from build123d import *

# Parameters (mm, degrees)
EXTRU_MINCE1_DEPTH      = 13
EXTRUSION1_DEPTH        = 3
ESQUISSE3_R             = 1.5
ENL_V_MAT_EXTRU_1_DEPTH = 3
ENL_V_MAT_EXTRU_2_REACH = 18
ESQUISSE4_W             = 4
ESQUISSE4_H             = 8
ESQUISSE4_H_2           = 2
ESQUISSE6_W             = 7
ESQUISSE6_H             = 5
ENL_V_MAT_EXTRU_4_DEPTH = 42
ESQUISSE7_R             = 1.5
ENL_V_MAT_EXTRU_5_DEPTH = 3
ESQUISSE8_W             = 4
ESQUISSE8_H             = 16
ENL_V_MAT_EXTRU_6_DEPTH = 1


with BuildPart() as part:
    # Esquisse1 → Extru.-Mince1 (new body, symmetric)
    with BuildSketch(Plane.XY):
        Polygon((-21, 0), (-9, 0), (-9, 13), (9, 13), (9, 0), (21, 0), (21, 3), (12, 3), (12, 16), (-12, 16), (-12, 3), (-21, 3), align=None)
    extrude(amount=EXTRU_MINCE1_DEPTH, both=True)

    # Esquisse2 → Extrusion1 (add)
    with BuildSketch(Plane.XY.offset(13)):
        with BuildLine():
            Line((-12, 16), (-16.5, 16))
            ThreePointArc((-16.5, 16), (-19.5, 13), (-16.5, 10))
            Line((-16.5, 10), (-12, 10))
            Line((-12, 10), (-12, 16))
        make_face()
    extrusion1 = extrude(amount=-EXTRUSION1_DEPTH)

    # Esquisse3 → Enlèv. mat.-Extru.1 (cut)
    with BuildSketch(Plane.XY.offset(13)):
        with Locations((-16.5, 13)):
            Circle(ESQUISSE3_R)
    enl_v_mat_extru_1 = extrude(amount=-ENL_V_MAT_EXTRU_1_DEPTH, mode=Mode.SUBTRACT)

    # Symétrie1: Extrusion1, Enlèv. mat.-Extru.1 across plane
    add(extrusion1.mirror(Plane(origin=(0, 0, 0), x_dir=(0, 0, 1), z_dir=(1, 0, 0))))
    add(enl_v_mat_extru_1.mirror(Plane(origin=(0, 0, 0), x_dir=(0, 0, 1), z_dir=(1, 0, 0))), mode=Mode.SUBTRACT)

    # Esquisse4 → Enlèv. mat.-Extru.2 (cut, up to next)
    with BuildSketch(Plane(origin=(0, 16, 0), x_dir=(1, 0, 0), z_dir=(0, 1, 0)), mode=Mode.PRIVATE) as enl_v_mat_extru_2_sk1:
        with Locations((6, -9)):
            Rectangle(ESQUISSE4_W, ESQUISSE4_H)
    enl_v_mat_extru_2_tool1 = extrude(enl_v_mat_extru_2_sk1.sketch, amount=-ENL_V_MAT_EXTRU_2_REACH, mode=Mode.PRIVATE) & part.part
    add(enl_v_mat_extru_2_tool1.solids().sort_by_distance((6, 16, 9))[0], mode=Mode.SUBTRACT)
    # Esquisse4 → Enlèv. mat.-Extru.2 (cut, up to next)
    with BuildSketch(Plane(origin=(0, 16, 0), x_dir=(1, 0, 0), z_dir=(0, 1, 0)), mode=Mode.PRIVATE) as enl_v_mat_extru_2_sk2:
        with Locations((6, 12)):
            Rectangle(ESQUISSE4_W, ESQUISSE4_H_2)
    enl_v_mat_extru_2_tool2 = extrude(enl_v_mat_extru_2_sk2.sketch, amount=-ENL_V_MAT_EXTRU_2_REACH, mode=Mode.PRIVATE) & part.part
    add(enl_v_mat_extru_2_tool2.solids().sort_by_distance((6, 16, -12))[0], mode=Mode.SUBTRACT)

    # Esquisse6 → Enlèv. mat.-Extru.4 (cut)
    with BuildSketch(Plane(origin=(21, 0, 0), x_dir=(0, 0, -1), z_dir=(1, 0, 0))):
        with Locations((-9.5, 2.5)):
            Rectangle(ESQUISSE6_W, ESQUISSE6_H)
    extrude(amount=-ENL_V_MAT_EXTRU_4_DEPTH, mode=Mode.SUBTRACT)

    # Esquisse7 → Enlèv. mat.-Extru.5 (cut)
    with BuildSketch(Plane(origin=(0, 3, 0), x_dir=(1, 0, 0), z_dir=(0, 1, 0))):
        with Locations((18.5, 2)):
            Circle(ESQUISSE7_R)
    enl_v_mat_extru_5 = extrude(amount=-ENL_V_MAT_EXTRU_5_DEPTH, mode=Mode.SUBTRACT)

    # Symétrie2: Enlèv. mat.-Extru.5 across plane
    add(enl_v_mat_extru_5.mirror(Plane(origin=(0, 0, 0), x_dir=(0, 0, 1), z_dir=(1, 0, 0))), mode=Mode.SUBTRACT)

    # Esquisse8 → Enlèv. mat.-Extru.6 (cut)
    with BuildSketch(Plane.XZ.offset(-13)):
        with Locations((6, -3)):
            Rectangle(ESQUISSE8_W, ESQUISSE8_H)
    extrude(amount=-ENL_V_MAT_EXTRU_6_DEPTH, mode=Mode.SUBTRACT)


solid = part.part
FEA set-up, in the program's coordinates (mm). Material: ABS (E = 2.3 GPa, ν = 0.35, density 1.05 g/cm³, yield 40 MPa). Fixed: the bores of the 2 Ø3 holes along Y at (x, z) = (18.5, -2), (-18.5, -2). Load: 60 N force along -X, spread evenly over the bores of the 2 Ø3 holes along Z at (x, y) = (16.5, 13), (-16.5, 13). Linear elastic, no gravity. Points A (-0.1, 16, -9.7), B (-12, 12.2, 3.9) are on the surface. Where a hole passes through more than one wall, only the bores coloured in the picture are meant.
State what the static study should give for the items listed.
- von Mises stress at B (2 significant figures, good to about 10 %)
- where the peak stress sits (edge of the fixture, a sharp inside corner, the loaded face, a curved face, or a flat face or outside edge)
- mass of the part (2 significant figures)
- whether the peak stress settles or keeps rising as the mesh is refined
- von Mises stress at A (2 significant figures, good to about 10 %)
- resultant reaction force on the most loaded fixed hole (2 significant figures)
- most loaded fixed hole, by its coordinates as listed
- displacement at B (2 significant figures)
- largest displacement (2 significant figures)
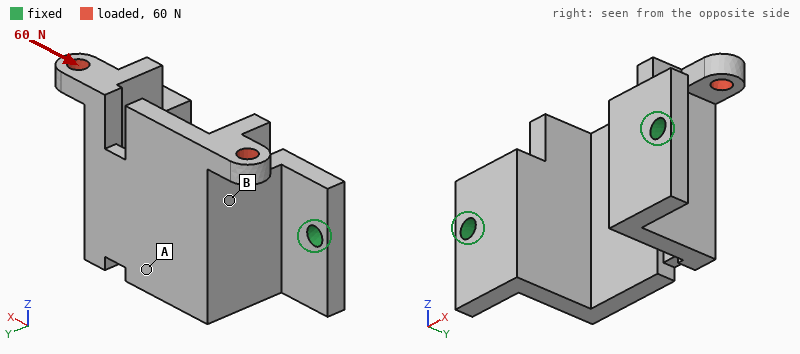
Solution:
5.9 MPa
a sharp inside corner
4.9 g
keeps rising
3.3 MPa
42 N
(-18.5, -2)
0.20 mm
0.53 mm
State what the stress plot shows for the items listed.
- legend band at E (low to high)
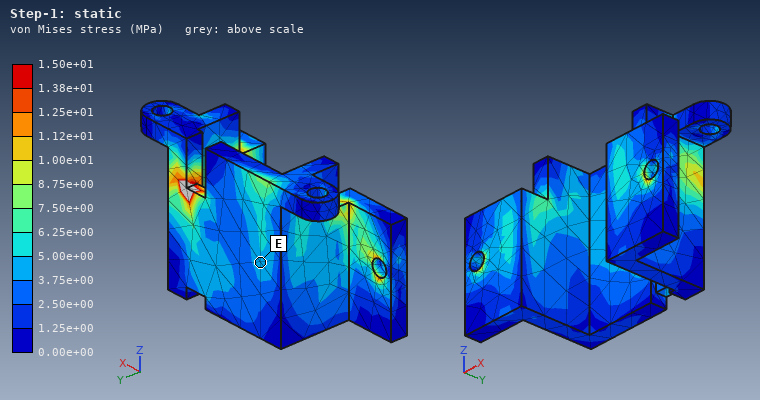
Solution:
3.75e+00 to 5.00e+00 MPa
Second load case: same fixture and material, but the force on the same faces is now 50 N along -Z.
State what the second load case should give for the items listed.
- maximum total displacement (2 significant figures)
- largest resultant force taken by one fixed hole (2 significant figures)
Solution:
0.59 mm
26 N
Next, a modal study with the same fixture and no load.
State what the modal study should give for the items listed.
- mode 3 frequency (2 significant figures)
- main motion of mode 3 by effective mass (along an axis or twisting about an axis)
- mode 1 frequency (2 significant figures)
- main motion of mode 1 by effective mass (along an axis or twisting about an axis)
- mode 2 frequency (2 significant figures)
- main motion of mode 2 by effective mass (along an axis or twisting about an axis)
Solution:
2300 Hz
along X
1100 Hz
along Z
1800 Hz
along X
